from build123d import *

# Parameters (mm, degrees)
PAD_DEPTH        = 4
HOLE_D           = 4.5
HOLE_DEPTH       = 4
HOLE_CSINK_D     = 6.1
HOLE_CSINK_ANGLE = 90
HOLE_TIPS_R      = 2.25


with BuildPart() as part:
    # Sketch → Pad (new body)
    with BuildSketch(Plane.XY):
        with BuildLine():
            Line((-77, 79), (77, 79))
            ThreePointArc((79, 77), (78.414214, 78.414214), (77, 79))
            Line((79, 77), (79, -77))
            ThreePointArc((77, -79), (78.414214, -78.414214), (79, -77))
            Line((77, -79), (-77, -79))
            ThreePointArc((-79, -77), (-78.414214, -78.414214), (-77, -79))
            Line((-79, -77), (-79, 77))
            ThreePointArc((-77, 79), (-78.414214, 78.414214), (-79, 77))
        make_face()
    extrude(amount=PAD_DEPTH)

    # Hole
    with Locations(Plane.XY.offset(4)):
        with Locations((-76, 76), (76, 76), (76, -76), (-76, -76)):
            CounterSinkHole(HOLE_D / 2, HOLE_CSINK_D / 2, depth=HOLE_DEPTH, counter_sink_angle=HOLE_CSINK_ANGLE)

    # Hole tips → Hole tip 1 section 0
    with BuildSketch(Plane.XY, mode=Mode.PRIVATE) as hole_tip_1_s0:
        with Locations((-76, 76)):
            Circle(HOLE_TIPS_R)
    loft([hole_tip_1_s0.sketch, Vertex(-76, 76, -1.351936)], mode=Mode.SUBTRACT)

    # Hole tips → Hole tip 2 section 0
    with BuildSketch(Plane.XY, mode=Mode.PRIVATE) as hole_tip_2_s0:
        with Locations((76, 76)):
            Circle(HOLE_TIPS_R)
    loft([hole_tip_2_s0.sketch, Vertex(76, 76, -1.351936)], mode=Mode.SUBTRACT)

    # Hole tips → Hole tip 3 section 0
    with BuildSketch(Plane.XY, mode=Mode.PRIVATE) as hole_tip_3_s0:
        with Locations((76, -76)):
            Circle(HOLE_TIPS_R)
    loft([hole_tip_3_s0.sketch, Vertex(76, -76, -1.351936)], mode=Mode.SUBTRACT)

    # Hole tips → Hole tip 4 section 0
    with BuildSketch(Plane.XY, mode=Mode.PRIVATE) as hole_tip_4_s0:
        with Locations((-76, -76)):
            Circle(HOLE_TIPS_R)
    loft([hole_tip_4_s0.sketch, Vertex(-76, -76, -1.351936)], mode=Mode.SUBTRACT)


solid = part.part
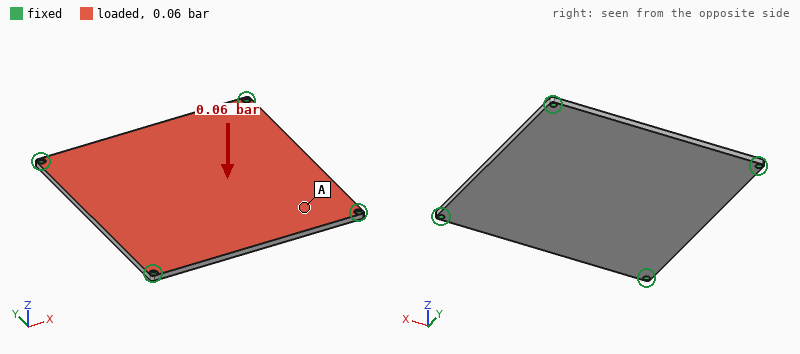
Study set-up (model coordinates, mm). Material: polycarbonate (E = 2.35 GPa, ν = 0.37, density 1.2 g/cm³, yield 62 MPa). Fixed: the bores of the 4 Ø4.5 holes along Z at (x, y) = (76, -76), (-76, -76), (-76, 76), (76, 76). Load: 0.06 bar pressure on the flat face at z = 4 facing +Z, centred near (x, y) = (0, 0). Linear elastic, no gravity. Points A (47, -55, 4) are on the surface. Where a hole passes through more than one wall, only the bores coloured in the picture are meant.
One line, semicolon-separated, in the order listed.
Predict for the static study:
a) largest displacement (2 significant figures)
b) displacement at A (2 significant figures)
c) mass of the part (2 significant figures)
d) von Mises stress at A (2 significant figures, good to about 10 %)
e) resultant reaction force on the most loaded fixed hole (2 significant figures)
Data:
2.4 mm; 1.1 mm; 120 g; 1.8 MPa; 40 N
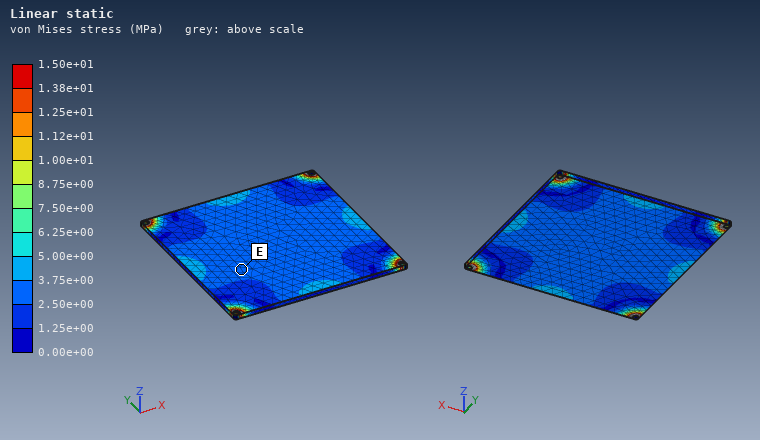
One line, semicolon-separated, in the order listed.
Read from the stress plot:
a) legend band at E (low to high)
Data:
2.50e+00 to 3.75e+00 MPa
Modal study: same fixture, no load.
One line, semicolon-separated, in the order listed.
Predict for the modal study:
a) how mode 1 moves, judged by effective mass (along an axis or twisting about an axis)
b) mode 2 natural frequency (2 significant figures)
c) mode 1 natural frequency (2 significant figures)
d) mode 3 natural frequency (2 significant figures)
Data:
along Z; 250 Hz; 130 Hz; 250 Hz
